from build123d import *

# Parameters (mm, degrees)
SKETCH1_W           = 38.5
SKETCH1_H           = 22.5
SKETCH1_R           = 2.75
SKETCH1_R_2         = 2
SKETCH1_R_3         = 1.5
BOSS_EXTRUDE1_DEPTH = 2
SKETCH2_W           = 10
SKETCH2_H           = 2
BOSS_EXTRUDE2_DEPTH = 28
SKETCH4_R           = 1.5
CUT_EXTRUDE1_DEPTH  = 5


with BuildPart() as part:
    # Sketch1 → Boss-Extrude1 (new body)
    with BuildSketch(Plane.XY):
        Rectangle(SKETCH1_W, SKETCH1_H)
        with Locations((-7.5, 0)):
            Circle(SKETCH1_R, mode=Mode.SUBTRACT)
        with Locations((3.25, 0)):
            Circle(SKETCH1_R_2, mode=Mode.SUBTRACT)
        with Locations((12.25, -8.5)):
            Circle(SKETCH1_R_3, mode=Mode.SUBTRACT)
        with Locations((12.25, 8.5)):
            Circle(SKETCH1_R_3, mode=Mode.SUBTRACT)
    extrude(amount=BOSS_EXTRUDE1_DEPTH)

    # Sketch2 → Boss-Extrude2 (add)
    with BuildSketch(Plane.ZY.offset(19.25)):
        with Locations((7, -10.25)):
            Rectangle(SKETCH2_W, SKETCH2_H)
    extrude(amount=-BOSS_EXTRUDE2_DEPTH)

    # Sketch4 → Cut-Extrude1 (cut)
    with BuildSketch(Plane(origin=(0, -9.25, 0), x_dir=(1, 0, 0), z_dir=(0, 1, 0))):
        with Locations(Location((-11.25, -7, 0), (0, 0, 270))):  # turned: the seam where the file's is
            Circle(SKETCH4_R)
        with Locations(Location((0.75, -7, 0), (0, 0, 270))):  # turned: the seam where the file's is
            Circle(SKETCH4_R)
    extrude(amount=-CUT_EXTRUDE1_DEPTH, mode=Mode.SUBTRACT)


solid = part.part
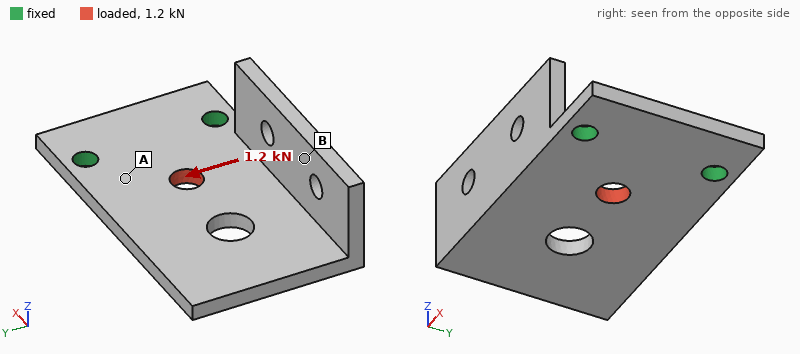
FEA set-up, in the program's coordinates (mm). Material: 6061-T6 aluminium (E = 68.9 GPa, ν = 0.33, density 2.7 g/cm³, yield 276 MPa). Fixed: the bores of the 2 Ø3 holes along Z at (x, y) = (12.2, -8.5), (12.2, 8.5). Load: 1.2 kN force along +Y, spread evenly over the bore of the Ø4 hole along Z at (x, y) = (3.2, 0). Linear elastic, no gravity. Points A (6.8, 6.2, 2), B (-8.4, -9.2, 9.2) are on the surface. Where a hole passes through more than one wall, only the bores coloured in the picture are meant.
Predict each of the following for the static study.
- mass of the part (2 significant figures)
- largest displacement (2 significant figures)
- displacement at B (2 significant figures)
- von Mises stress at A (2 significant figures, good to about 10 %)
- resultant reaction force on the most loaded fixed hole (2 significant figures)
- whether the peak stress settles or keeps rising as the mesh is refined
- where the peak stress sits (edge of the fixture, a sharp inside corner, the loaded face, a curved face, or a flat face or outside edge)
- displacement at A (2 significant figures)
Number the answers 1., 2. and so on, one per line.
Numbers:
1. 5.8 g
2. 23 µm
3. 19 µm
4. 54 MPa
5. 820 N
6. keeps rising
7. edge of the fixture
8. 7.0 µm
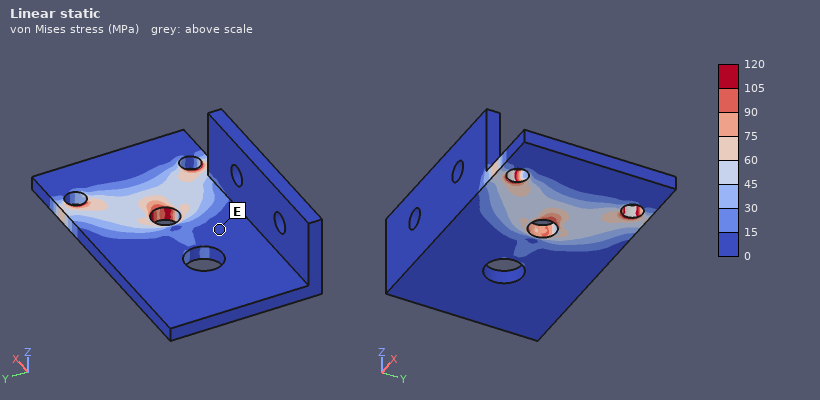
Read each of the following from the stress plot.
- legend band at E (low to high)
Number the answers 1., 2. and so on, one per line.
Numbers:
1. 0 to 15 MPa
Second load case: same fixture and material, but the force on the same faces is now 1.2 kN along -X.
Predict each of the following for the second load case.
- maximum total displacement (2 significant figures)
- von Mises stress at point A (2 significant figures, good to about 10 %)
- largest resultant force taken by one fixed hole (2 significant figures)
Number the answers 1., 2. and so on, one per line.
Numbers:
1. 8.5 µm
2. 32 MPa
3. 610 N
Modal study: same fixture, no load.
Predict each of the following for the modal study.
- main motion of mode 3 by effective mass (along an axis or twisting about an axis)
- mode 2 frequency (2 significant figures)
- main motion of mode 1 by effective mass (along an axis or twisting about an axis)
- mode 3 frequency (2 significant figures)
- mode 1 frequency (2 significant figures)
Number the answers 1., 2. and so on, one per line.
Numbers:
1. along Y
2. 3800 Hz
3. along Z
4. 8500 Hz
5. 1600 Hz
